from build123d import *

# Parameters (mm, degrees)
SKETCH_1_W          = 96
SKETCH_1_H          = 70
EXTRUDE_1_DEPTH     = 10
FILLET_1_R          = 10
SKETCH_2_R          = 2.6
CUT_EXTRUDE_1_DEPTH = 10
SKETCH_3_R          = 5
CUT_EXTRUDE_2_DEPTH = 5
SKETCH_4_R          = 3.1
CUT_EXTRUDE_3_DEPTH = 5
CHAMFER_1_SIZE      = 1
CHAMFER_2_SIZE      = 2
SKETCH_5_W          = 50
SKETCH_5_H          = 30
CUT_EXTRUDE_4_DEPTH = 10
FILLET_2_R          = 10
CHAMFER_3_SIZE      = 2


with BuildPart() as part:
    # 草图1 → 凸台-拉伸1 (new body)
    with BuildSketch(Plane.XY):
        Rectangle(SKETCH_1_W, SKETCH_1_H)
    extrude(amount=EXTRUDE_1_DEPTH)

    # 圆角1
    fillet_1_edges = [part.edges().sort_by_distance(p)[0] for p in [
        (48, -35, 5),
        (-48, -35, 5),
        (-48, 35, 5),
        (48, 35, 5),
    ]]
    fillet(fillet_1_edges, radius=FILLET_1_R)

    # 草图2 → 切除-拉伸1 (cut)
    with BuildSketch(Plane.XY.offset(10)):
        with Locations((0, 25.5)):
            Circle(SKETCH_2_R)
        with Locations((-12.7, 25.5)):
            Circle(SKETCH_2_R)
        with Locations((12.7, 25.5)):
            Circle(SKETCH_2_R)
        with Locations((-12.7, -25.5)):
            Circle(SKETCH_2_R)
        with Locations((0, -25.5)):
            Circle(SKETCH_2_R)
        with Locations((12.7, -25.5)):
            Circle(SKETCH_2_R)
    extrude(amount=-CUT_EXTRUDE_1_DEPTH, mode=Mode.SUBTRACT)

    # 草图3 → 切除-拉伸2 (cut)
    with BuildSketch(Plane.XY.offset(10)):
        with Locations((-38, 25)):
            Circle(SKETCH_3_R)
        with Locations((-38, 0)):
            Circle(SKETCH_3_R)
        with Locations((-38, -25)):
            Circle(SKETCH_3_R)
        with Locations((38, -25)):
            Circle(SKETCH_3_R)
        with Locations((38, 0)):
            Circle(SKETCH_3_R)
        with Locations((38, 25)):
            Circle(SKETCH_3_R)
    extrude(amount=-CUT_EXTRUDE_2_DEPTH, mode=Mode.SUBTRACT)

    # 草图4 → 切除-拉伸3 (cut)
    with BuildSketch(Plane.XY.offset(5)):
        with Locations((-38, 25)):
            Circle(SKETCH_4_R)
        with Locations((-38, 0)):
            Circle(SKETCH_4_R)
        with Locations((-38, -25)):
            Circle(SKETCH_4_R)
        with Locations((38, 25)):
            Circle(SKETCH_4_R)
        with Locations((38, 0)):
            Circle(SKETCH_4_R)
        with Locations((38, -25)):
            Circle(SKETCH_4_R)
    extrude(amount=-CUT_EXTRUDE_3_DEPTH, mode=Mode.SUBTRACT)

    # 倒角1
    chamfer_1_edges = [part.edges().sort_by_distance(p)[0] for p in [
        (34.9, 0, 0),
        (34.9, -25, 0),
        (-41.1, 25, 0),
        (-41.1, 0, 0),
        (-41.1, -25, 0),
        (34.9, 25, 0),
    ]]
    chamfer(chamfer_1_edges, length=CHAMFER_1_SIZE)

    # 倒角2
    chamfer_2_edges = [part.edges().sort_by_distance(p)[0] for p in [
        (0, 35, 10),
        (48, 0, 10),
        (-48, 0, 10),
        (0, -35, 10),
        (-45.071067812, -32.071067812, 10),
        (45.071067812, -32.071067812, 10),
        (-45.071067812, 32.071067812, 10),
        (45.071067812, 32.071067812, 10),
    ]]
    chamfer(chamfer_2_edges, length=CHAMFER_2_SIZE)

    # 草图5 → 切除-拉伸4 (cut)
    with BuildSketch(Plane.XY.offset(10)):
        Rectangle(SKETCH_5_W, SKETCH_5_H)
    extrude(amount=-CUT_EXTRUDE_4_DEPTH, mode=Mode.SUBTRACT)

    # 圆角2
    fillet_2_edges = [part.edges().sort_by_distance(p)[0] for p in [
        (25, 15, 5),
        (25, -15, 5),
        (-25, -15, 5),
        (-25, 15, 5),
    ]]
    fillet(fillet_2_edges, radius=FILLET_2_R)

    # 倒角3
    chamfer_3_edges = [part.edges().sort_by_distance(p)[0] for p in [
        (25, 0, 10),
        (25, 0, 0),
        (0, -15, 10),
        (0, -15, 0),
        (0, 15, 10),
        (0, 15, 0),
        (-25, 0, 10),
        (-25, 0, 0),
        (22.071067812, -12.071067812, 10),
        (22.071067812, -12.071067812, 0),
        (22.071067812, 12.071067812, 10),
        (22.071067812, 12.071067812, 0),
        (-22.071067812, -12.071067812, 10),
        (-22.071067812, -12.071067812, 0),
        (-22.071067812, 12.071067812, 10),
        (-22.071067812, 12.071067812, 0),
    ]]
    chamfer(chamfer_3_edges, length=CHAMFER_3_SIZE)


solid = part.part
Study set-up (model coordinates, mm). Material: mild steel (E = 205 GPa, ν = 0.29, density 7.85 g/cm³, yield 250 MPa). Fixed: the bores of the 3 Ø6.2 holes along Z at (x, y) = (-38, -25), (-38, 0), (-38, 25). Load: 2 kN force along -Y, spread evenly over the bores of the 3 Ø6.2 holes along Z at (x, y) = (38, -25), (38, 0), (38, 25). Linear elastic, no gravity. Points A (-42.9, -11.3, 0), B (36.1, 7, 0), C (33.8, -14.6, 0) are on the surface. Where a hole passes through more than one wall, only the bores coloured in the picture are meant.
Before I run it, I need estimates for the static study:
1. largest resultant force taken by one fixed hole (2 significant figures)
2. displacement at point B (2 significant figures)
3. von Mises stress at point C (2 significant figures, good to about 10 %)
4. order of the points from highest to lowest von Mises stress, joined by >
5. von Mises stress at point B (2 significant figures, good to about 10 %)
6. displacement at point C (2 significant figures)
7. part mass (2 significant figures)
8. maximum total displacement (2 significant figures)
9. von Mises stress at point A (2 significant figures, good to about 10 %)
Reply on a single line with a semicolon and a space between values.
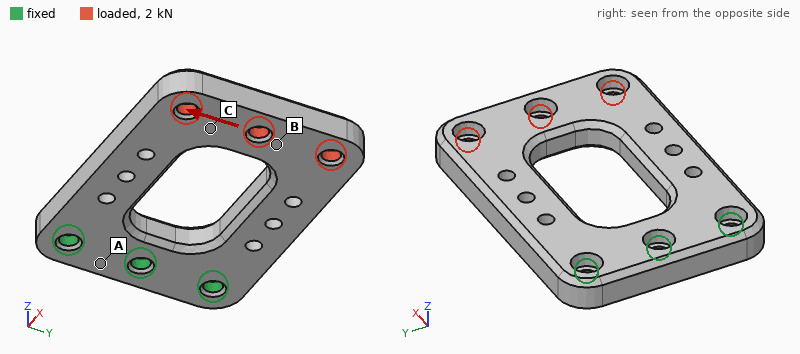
2.8 kN; 34 µm; 16 MPa; B > C > A; 27 MPa; 34 µm; 360 g; 40 µm; 7.1 MPa
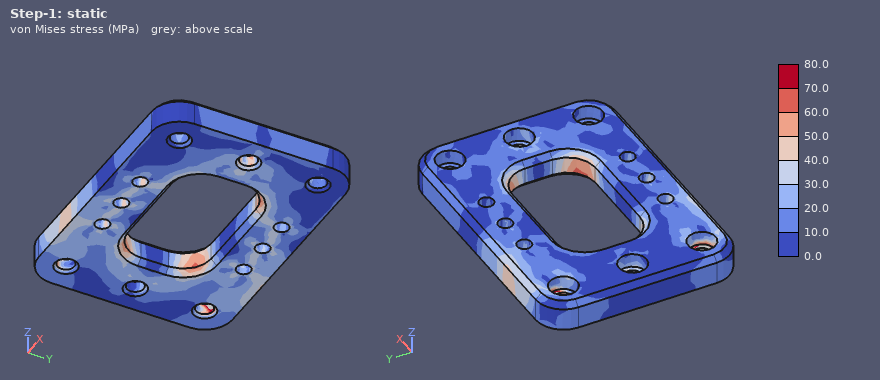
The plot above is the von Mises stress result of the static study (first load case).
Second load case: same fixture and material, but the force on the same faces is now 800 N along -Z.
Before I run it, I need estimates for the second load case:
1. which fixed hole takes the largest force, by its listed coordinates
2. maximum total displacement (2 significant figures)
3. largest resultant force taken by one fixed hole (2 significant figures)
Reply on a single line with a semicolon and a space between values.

(-38, 0); 0.28 mm; 480 N
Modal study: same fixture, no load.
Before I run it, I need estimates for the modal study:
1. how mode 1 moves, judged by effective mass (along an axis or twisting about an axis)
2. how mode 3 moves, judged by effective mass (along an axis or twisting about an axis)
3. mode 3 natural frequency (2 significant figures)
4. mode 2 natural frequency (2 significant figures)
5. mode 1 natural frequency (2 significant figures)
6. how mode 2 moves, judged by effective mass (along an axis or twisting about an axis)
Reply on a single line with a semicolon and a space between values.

along Z; along Y; 3300 Hz; 2300 Hz; 810 Hz; twisting about X
